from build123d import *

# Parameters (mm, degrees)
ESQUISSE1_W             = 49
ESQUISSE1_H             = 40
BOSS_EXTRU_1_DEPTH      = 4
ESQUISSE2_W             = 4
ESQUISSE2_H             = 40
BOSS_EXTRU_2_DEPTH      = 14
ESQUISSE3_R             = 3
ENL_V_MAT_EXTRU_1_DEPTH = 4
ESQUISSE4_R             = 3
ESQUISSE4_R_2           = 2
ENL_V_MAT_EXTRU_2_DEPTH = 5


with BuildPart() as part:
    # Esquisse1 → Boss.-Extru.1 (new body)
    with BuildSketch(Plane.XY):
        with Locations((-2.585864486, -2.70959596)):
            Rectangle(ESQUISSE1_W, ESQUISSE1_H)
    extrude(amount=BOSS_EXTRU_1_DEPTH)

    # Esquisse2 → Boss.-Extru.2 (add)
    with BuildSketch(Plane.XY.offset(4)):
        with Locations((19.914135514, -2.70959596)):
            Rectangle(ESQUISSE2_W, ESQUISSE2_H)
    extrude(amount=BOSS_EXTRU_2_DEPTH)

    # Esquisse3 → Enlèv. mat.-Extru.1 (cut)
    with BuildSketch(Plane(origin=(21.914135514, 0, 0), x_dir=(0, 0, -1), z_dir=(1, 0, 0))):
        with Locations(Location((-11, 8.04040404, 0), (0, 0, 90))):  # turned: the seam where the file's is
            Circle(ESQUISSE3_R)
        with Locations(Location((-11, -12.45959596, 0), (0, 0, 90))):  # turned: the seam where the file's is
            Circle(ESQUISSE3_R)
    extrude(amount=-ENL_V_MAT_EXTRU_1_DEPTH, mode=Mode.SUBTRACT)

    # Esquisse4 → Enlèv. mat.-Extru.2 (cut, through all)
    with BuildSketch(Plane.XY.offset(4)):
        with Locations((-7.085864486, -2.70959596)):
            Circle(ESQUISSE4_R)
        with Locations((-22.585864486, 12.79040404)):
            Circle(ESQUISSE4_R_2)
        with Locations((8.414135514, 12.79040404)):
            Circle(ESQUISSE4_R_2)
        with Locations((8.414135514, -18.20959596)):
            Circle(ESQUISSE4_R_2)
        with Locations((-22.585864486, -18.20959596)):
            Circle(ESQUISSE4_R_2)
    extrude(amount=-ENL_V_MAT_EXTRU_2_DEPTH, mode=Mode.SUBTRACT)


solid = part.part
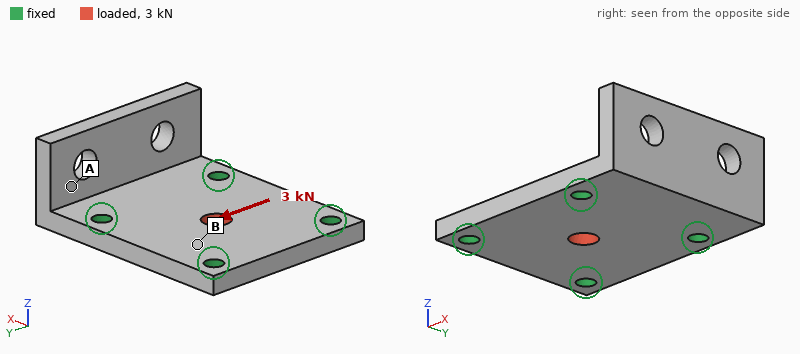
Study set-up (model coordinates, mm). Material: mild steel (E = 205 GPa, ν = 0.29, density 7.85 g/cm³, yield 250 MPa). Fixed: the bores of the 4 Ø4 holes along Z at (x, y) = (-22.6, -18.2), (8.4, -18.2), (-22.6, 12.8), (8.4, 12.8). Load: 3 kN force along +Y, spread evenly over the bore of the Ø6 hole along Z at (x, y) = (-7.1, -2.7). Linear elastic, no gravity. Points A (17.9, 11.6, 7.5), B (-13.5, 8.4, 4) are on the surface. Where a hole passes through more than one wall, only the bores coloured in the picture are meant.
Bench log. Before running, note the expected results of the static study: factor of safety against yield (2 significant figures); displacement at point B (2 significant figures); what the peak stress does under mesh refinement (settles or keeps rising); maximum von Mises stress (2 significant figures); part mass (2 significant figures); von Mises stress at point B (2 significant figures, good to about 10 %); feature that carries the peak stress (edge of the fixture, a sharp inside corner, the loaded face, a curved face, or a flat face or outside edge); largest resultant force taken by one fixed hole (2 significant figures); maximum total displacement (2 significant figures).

3.6
1.3 µm
settles
69 MPa
75 g
19 MPa
the loaded face
850 N
2.7 µm
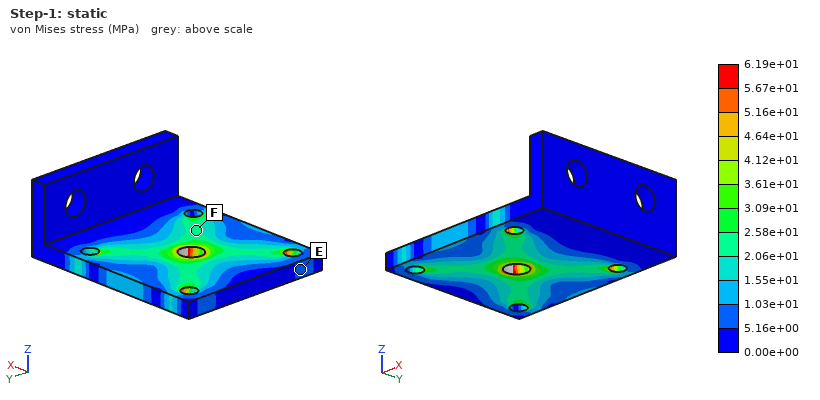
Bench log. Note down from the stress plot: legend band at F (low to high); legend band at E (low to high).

2.06e+01 to 2.58e+01 MPa
5.16e+00 to 1.03e+01 MPa
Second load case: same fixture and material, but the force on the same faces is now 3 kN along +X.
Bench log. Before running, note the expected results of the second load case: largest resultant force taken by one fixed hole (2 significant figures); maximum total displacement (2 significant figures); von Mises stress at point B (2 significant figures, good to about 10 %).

850 N
2.7 µm
16 MPa
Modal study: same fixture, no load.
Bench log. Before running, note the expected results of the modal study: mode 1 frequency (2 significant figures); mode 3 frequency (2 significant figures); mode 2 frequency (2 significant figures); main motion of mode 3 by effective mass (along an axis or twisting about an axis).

5800 Hz
15 kHz
10 kHz
along Z
